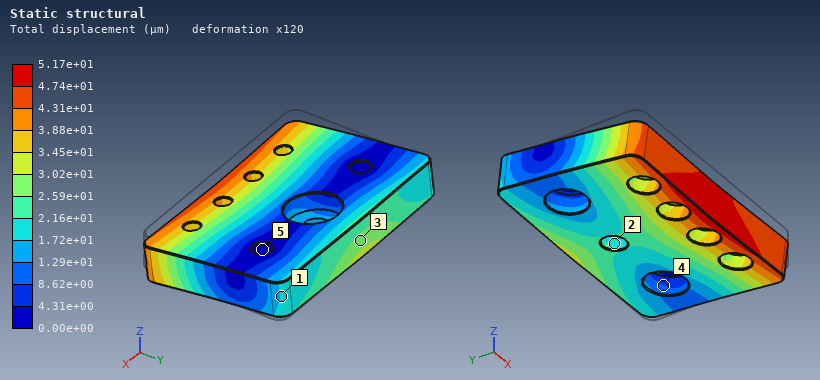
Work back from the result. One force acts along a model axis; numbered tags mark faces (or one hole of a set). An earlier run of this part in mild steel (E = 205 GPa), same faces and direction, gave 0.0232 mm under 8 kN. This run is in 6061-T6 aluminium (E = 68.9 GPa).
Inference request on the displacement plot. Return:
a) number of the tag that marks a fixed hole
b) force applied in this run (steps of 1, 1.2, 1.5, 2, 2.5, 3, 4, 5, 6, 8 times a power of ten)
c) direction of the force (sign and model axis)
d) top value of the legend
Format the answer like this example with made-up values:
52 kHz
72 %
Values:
5
6 kN
+Y
5.17e+01 µm
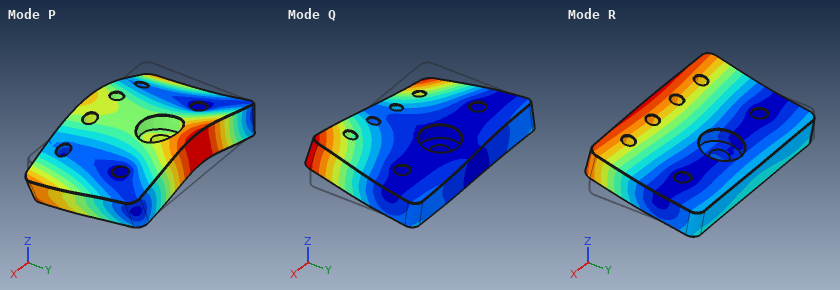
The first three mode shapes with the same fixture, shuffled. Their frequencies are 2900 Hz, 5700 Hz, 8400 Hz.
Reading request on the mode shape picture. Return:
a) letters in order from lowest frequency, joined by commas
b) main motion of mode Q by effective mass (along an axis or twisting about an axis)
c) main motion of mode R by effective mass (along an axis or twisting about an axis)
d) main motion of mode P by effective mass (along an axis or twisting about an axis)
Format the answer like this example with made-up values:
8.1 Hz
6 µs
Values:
R, Q, P
twisting about Y
along Z
along Z
